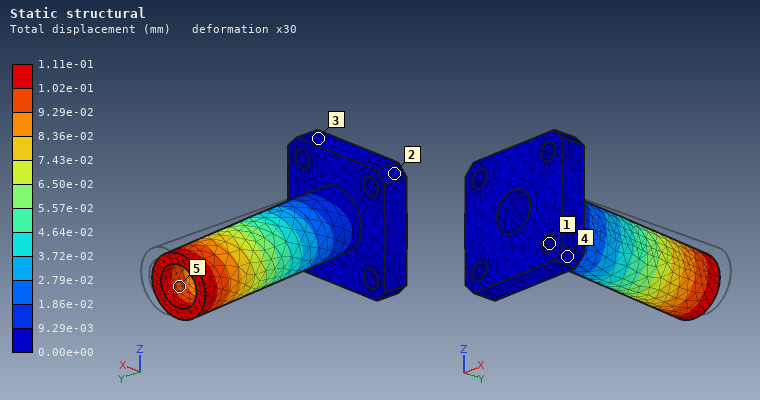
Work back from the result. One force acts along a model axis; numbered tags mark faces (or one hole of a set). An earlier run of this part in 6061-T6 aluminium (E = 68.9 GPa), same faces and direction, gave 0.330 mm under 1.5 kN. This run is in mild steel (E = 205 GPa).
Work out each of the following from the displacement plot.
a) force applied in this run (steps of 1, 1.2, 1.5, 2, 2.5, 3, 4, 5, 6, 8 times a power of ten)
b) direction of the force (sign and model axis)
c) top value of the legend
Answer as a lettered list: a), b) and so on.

a) 1.5 kN
b) -X
c) 1.11e-01 mm
